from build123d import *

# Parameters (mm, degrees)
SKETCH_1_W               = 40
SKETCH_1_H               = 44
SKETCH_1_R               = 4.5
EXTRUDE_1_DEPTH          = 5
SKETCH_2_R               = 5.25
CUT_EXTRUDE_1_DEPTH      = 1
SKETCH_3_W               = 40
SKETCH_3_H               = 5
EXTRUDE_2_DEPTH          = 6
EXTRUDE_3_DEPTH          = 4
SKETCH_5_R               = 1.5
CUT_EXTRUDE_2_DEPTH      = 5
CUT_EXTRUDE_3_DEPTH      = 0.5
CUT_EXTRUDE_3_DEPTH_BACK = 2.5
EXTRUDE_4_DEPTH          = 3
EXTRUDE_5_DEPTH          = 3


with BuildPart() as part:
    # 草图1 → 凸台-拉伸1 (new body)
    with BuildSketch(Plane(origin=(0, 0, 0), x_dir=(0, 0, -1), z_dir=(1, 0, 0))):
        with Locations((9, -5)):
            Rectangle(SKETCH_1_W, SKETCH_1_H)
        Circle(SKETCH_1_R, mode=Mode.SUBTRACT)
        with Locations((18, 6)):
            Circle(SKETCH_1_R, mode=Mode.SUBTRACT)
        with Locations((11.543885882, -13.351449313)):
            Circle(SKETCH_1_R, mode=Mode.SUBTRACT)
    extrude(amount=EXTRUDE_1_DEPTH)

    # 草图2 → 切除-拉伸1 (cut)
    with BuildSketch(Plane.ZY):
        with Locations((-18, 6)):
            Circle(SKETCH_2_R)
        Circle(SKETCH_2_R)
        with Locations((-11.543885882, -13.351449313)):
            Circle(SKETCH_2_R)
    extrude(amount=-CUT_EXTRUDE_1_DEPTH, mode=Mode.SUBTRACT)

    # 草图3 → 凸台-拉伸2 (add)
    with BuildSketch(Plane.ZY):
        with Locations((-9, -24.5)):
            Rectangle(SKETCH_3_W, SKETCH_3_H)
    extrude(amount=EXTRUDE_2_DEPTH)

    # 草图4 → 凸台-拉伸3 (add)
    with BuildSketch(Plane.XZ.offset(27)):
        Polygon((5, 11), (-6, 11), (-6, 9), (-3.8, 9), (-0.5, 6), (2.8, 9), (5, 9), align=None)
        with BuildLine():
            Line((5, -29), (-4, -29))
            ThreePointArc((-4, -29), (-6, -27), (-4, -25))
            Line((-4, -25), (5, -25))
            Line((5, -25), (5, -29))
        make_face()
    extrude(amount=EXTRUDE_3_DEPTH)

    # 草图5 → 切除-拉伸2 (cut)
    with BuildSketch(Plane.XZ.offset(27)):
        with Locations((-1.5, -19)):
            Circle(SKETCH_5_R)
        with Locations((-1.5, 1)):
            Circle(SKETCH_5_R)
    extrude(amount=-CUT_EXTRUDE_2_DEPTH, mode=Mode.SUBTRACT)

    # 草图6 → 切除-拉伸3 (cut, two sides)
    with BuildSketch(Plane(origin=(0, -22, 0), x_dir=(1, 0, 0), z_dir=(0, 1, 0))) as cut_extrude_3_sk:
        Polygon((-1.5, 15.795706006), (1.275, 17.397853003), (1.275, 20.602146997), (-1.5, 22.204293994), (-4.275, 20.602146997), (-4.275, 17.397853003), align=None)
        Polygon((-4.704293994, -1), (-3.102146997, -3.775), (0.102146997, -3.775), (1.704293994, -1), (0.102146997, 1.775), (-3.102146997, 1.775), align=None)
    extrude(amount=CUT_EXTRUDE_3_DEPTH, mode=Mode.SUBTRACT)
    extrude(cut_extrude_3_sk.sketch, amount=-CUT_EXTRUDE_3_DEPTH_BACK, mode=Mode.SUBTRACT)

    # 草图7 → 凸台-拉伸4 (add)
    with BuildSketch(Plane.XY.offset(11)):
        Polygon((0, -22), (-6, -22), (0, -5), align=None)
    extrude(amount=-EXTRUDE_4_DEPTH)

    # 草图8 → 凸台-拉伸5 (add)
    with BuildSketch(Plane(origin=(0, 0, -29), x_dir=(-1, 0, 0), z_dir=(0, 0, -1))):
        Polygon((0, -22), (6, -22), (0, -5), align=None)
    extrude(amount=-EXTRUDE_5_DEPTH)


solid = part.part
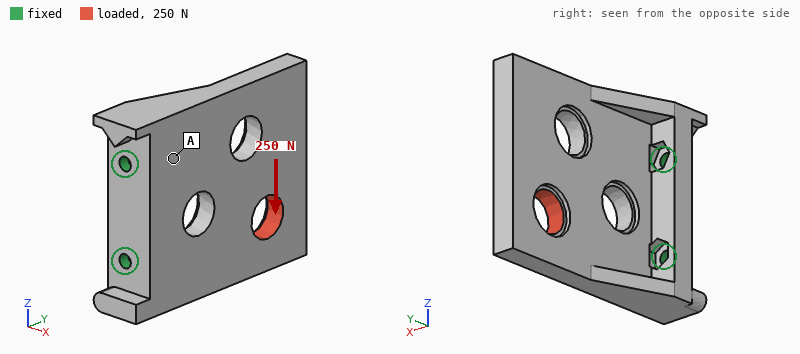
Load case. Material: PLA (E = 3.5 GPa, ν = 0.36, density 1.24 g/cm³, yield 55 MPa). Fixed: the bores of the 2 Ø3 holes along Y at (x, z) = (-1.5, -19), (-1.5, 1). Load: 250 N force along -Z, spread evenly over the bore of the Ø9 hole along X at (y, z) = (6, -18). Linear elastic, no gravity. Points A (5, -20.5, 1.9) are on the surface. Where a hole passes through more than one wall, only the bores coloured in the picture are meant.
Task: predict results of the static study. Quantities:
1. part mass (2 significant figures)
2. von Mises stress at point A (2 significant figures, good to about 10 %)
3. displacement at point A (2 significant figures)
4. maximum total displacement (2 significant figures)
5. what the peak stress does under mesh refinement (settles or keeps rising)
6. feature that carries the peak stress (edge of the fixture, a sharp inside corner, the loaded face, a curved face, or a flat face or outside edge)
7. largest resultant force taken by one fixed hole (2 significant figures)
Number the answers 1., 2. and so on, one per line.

1. 12 g
2. 5.5 MPa
3. 0.086 mm
4. 0.44 mm
5. keeps rising
6. edge of the fixture
7. 390 N
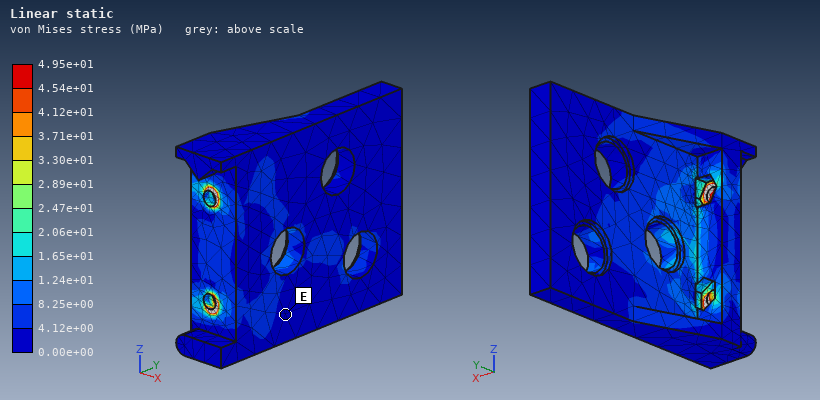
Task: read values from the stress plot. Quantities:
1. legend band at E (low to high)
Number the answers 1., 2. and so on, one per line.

1. 0.00e+00 to 4.12e+00 MPa
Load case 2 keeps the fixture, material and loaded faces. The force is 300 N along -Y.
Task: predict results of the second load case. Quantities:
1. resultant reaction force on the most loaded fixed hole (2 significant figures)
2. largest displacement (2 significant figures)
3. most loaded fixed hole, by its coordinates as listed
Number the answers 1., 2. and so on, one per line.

1. 270 N
2. 0.67 mm
3. (-1.5, -19)
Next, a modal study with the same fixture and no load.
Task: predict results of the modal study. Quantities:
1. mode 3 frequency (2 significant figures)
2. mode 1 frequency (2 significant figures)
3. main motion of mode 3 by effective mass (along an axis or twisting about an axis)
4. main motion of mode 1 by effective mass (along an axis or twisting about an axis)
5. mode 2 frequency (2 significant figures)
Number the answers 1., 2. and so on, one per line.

1. 2000 Hz
2. 550 Hz
3. along Z
4. along X
5. 1400 Hz
